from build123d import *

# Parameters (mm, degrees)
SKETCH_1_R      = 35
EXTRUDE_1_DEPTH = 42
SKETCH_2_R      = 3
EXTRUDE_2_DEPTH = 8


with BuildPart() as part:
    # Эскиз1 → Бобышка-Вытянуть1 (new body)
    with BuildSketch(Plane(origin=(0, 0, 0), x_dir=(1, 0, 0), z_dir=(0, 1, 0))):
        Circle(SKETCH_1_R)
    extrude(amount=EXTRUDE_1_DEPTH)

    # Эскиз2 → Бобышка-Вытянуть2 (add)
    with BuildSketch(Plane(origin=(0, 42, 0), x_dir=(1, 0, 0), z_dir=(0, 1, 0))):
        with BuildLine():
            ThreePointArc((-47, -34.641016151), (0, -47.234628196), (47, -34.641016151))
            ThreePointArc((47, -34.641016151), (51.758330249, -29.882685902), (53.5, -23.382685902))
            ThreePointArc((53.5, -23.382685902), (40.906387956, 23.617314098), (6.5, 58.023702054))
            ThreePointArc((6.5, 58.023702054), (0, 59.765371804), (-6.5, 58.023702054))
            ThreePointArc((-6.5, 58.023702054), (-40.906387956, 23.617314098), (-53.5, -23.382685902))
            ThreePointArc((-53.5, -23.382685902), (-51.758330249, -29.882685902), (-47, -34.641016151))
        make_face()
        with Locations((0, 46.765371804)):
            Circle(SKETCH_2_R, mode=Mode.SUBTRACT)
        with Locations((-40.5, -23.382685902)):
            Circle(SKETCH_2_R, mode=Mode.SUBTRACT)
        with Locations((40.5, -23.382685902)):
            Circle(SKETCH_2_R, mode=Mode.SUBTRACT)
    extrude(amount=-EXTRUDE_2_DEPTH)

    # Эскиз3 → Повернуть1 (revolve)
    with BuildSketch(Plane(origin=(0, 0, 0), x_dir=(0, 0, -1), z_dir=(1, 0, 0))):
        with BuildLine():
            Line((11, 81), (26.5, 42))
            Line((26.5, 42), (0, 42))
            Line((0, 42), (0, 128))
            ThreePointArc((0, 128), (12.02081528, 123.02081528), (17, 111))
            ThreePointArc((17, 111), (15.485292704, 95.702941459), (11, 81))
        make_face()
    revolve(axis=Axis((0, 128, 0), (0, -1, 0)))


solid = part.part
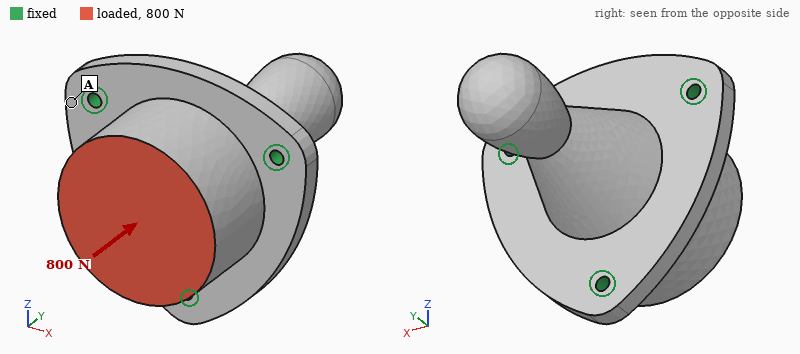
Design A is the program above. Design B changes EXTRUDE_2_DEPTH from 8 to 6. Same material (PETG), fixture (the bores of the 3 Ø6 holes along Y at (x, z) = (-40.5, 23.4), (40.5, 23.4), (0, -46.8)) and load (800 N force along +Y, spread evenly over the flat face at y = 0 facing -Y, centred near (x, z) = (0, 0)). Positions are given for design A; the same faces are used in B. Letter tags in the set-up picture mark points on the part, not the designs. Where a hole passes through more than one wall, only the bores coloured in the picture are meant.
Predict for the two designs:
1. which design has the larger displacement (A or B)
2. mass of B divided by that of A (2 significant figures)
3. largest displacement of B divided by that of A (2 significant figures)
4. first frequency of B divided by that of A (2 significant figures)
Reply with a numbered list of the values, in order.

1. B
2. 0.97
3. 1.6
4. 0.86
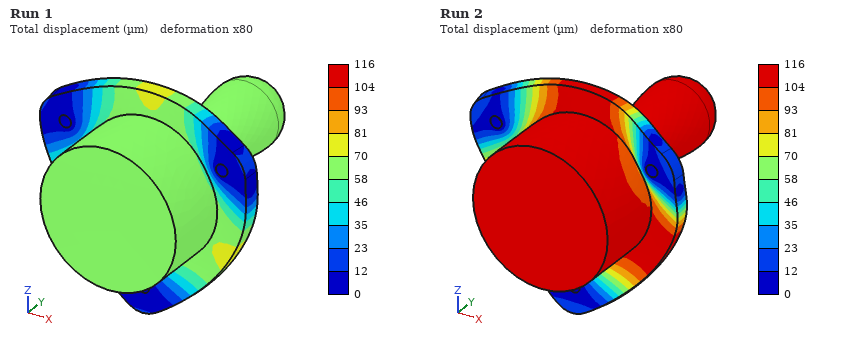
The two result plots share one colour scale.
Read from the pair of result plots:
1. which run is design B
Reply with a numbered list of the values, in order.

1. Run 2
